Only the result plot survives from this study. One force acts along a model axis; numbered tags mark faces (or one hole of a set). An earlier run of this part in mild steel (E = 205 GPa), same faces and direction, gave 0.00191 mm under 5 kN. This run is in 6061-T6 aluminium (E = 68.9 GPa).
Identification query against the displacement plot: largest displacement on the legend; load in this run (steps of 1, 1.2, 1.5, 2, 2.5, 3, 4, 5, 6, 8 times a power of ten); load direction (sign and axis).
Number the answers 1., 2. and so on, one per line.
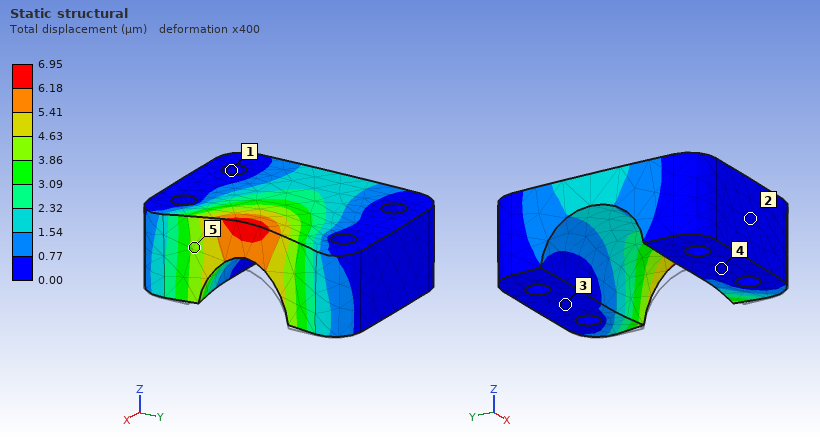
1. 6.95 µm
2. 6 kN
3. -X
